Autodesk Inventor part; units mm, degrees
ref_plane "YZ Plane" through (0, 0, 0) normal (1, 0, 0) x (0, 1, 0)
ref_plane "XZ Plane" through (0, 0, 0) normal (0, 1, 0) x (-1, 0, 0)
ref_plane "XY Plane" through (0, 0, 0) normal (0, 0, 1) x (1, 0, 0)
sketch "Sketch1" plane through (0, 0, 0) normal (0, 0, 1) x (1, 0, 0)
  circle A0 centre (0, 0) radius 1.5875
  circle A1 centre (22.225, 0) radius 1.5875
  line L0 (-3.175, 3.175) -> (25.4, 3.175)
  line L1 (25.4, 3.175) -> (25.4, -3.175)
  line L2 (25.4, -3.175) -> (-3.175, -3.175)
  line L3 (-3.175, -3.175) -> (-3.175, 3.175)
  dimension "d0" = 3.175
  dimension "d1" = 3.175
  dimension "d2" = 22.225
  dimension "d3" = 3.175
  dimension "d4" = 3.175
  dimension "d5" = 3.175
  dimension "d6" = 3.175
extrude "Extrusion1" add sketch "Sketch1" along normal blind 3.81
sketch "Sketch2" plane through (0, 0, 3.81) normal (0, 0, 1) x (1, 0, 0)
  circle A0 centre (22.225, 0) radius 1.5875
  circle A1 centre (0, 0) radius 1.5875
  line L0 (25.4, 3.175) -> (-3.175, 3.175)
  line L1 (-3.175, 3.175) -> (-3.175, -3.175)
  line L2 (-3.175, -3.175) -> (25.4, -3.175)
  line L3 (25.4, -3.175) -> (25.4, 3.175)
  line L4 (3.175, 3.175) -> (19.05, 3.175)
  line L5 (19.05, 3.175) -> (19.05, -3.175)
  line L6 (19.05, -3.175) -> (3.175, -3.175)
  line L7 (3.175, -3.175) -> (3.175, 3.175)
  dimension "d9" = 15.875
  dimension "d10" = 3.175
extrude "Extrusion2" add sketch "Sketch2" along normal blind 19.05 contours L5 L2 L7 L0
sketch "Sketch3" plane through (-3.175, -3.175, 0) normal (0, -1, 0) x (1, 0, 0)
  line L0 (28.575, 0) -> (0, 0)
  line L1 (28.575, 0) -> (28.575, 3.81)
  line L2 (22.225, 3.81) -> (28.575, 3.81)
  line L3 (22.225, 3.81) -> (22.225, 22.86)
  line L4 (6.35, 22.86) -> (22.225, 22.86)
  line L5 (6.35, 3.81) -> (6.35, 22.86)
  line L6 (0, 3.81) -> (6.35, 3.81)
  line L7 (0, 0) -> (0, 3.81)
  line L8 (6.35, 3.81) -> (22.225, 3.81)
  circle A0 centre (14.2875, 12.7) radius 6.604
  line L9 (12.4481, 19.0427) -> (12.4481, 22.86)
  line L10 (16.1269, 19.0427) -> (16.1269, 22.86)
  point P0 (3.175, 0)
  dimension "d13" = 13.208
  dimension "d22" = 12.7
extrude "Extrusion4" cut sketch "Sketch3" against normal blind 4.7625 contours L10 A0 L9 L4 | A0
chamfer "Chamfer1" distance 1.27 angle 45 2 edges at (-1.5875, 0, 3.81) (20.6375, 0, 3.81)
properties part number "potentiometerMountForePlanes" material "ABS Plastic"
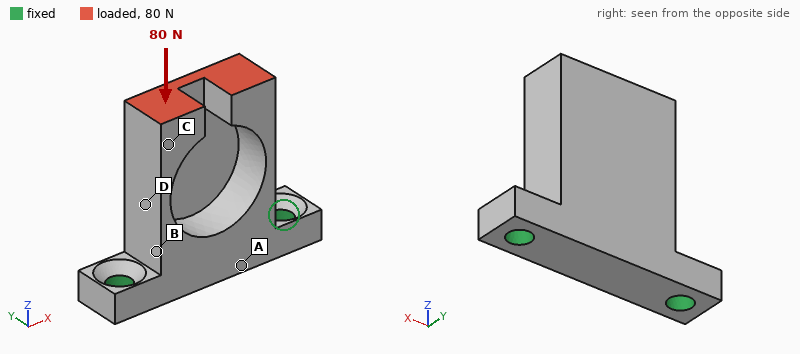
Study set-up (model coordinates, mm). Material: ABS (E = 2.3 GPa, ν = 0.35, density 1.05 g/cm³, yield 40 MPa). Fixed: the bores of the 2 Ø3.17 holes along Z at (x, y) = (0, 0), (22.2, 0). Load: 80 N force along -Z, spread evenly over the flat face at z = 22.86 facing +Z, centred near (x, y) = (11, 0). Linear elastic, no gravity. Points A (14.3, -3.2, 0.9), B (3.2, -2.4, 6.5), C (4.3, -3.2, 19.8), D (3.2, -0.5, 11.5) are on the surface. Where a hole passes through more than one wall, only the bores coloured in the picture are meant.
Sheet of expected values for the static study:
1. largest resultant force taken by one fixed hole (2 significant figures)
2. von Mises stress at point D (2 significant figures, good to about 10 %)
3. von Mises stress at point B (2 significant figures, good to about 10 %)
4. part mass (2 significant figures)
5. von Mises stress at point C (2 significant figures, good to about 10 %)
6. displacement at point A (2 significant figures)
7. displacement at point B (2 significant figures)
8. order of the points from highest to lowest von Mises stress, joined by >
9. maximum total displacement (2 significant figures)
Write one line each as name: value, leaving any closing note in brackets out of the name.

largest resultant force taken by one fixed hole: 45 N
von Mises stress at point D: 2.8 MPa
von Mises stress at point B: 3.7 MPa
part mass: 1.9 g
von Mises stress at point C: 1.9 MPa
displacement at point A: 14 µm
displacement at point B: 15 µm
order of the points from highest to lowest von Mises stress, joined by >: B > D > C > A
maximum total displacement: 57 µm
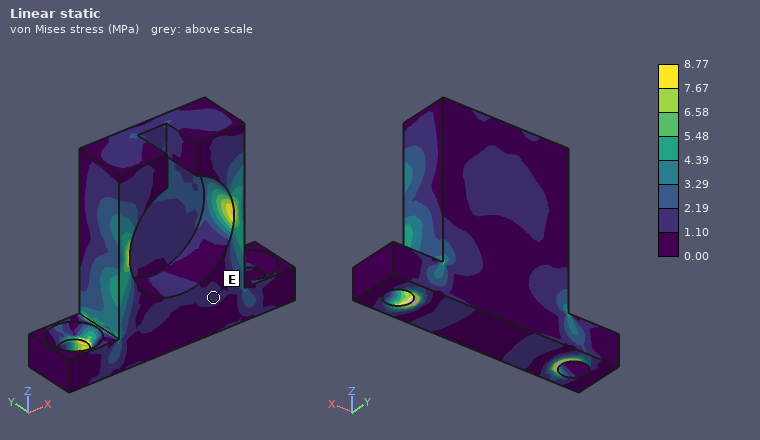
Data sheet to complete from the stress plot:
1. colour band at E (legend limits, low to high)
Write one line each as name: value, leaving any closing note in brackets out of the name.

colour band at E: 1.10 to 2.19 MPa
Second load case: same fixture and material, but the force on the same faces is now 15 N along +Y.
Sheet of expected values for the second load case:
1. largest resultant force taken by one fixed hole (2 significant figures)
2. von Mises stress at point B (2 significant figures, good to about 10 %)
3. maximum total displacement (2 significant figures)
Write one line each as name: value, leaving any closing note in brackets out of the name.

largest resultant force taken by one fixed hole: 8.5 N
von Mises stress at point B: 5.5 MPa
maximum total displacement: 0.37 mm
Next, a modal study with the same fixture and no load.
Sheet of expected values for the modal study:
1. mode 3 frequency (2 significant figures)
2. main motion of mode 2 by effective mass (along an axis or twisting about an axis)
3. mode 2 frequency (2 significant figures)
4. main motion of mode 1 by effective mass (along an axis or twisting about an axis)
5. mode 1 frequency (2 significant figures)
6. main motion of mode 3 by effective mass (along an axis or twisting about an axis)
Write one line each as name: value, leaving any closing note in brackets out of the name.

mode 3 frequency: 5500 Hz
main motion of mode 2 by effective mass: along X
mode 2 frequency: 3200 Hz
main motion of mode 1 by effective mass: along Y
mode 1 frequency: 1500 Hz
main motion of mode 3 by effective mass: along X
